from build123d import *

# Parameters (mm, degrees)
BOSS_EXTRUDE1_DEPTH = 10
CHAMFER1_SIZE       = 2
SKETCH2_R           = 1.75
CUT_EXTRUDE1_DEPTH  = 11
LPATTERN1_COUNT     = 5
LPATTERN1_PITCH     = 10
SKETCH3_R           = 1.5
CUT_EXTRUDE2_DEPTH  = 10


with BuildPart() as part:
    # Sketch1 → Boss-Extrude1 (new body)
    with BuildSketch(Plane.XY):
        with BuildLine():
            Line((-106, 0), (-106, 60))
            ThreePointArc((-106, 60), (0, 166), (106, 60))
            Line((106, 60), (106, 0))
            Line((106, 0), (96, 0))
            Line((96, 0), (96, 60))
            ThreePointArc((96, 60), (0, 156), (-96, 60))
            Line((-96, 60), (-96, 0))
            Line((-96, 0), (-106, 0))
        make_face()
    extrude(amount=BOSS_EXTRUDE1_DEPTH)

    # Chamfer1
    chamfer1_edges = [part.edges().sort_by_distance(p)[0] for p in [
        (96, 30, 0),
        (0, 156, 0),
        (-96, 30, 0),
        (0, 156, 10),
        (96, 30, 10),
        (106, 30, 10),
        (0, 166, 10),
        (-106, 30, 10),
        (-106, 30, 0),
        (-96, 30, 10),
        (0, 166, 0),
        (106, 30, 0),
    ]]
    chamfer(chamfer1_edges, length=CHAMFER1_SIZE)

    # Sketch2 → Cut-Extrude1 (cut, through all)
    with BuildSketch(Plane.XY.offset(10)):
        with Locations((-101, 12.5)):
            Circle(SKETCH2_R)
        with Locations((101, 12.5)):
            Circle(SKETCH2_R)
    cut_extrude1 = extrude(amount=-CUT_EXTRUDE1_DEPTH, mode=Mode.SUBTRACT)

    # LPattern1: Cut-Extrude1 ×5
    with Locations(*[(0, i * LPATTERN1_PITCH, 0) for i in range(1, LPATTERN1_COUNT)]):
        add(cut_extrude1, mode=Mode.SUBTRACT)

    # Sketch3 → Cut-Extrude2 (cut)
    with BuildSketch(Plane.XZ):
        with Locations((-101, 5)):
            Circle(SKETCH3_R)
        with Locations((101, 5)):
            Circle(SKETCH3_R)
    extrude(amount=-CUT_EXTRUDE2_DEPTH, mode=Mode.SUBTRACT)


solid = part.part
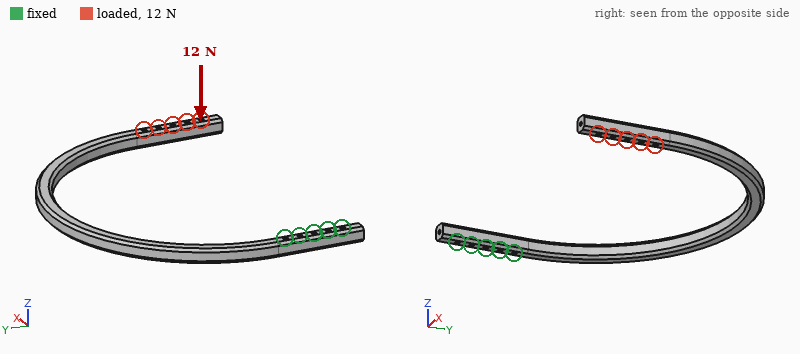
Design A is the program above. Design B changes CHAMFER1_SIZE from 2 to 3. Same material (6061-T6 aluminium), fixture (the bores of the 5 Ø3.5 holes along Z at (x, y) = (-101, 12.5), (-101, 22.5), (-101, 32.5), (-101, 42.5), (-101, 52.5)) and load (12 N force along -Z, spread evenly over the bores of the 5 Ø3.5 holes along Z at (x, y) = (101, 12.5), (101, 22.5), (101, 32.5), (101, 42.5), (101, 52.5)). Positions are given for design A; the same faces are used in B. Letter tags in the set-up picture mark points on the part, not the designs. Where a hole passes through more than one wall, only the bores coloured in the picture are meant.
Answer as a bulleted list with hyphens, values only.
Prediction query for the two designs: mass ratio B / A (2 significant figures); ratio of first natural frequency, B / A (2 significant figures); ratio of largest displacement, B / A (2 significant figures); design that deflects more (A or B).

- 0.89
- 0.96
- 1.2
- B
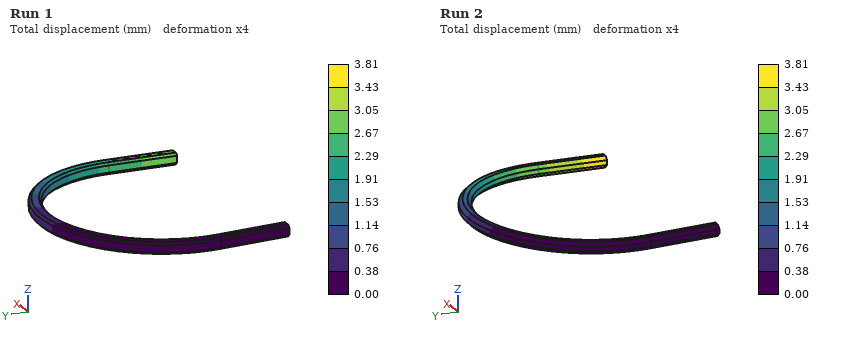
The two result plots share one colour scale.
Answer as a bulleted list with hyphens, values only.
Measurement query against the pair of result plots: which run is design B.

- Run 2
